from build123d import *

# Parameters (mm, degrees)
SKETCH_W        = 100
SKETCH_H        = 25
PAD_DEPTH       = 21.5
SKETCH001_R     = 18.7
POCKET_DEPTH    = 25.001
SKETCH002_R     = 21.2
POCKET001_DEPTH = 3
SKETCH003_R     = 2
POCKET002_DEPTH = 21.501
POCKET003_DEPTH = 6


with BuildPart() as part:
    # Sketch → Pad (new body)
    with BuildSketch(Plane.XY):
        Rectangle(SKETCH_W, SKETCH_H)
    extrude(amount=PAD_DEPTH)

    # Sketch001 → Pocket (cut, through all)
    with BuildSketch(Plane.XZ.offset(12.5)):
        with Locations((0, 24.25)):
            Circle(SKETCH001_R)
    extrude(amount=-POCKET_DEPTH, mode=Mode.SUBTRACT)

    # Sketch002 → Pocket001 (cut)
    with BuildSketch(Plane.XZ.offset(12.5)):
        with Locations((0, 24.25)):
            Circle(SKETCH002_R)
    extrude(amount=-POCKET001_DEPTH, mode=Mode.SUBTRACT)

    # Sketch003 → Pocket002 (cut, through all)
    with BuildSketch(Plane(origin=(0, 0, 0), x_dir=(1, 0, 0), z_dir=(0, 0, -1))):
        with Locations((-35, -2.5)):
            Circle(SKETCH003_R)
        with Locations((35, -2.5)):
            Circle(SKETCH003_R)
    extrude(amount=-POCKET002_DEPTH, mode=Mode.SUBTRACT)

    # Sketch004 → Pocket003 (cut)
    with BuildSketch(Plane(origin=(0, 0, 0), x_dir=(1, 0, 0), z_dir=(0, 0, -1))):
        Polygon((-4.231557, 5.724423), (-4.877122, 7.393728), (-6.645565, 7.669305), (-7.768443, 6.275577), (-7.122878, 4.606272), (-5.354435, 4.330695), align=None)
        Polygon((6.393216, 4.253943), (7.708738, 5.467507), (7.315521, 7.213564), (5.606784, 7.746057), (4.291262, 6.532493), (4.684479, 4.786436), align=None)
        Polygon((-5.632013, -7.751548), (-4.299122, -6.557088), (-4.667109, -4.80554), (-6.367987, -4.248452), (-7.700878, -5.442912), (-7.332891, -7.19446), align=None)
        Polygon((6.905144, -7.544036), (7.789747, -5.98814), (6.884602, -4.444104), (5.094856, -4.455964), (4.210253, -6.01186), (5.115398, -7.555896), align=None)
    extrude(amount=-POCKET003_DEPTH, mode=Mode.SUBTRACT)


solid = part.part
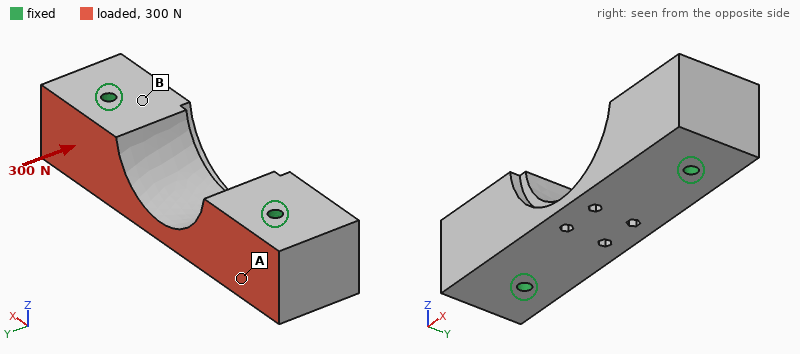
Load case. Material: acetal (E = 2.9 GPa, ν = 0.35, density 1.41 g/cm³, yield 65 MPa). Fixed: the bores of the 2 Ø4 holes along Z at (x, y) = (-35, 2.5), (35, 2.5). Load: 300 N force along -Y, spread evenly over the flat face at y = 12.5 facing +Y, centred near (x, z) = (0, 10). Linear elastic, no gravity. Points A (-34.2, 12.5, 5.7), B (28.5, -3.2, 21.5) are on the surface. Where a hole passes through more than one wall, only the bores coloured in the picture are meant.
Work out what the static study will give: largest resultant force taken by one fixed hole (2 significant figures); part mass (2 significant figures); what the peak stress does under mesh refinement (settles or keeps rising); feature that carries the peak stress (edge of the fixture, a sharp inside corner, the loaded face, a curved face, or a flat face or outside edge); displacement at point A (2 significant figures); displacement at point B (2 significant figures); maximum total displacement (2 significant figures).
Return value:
150 N
58 g
keeps rising
edge of the fixture
3.4 µm
3.3 µm
15 µm
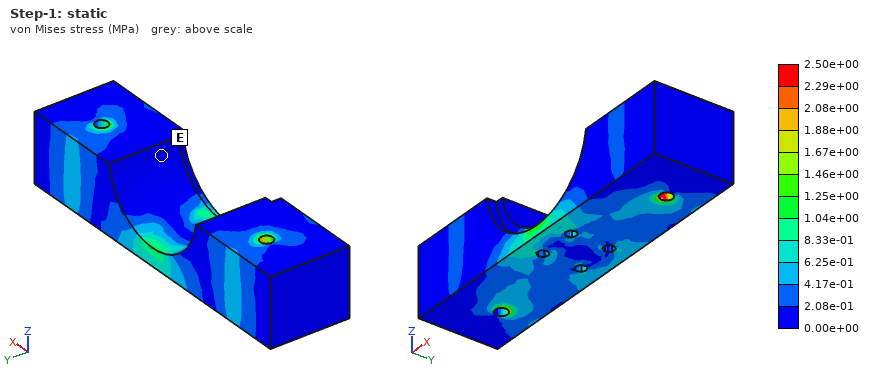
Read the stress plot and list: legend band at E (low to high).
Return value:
0.00e+00 to 2.08e-01 MPa
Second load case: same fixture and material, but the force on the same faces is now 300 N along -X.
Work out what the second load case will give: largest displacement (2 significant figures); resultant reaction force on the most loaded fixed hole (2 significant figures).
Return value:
7.9 µm
150 N
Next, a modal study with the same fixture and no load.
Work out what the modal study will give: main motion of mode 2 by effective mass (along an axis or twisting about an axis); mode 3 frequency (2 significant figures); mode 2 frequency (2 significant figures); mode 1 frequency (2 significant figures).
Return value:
along Z
5300 Hz
4700 Hz
2900 Hz
